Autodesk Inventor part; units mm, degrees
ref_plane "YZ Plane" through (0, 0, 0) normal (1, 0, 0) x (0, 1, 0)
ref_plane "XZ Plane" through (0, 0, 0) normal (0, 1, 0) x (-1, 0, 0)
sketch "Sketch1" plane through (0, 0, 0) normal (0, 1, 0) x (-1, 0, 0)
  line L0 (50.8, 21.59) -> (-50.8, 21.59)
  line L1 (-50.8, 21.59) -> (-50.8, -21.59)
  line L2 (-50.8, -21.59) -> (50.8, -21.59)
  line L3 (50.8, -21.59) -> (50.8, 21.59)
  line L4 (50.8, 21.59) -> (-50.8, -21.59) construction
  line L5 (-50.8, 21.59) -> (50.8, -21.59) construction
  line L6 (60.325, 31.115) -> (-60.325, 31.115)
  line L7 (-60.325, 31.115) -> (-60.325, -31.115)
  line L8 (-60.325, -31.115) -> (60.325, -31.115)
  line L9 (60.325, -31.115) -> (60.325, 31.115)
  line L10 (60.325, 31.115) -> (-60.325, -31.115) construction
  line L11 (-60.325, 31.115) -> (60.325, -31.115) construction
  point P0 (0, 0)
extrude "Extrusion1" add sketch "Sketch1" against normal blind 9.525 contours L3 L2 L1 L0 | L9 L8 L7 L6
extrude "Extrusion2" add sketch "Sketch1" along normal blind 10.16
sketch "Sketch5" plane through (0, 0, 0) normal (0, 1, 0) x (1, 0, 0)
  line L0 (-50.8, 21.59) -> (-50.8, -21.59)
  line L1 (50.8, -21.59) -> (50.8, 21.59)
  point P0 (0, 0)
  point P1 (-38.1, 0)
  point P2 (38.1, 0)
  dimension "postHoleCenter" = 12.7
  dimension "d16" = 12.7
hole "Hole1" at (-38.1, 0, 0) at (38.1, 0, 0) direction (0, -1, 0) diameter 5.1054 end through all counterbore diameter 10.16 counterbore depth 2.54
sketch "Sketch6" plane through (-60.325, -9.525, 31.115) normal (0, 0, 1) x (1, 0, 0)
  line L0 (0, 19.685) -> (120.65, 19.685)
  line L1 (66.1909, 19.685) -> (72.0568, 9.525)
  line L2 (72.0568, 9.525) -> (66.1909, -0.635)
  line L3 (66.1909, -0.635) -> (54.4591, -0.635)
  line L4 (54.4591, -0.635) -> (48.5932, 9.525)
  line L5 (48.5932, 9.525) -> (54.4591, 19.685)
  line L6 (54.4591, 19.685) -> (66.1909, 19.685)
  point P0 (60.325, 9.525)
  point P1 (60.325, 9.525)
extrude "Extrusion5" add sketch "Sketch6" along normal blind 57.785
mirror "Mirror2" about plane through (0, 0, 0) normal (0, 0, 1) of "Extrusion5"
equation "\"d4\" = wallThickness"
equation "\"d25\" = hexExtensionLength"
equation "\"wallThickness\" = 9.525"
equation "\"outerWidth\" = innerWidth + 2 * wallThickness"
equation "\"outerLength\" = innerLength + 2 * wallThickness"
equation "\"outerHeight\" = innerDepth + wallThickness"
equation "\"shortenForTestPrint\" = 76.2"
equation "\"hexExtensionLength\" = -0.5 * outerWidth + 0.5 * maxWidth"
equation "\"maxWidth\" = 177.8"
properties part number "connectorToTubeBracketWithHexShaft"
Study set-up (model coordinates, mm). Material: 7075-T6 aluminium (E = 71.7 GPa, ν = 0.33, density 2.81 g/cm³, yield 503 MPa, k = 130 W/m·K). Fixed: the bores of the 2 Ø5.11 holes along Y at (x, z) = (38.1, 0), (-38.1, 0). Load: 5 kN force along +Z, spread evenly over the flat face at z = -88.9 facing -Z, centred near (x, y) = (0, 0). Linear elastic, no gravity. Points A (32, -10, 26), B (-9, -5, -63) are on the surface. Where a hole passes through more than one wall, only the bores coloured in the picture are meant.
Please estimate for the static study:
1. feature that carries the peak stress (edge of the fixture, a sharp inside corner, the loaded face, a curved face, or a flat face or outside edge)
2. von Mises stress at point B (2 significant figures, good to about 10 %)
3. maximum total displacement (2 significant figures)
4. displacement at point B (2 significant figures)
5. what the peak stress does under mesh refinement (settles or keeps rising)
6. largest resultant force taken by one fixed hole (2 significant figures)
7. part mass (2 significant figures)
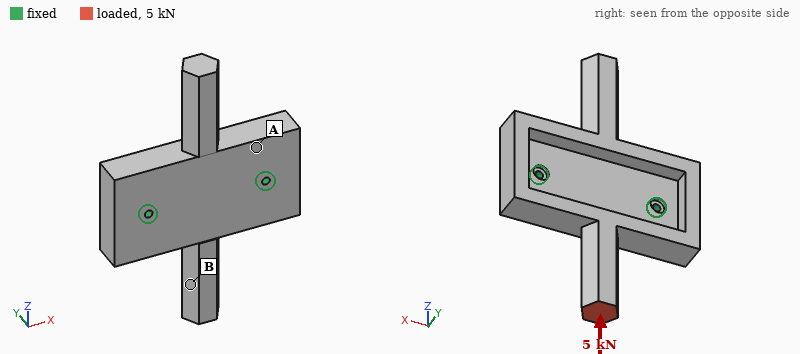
edge of the fixture
14 MPa
0.19 mm
0.12 mm
keeps rising
2.5 kN
400 g
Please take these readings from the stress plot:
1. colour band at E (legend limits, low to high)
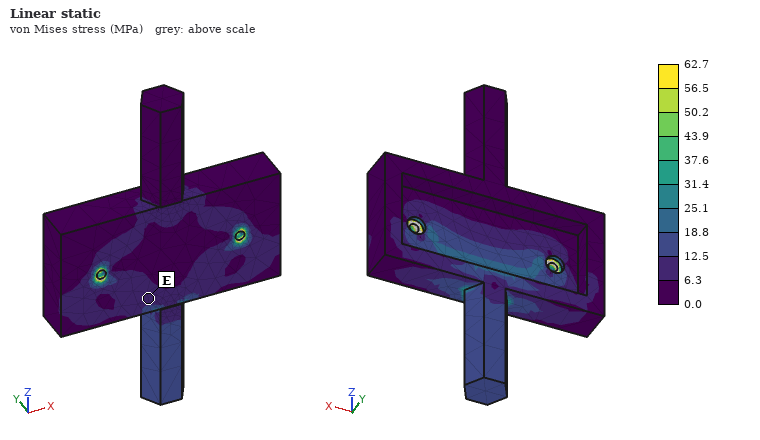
6.3 to 12.5 MPa
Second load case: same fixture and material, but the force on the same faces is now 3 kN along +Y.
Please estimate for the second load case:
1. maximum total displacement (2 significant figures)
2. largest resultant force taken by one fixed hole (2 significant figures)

2.1 mm
1.6 kN
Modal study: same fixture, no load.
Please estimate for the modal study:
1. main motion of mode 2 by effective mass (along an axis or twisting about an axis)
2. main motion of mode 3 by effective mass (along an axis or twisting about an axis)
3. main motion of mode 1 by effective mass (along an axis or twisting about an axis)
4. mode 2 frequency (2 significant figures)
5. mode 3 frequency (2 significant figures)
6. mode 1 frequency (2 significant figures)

along Y
twisting about Y
twisting about X
1600 Hz
3100 Hz
950 Hz
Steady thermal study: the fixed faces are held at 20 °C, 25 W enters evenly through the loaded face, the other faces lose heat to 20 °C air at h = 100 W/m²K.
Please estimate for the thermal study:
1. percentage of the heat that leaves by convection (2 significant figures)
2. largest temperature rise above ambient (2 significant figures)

55 %
33 K
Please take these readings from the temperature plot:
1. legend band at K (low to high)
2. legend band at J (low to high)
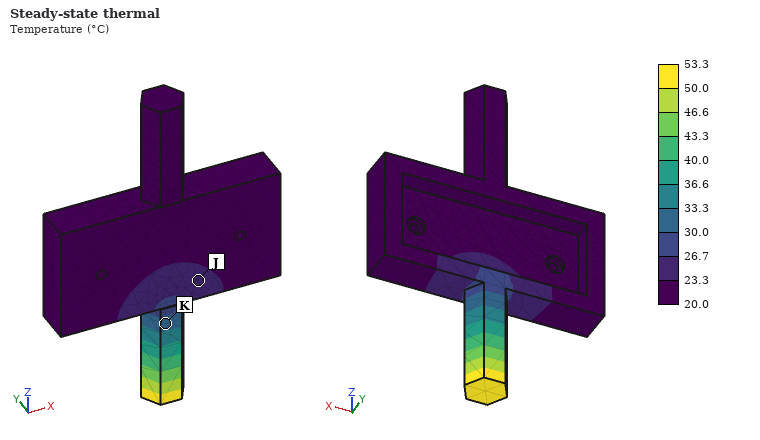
30.0 to 33.3 °C
23.3 to 26.7 °C
